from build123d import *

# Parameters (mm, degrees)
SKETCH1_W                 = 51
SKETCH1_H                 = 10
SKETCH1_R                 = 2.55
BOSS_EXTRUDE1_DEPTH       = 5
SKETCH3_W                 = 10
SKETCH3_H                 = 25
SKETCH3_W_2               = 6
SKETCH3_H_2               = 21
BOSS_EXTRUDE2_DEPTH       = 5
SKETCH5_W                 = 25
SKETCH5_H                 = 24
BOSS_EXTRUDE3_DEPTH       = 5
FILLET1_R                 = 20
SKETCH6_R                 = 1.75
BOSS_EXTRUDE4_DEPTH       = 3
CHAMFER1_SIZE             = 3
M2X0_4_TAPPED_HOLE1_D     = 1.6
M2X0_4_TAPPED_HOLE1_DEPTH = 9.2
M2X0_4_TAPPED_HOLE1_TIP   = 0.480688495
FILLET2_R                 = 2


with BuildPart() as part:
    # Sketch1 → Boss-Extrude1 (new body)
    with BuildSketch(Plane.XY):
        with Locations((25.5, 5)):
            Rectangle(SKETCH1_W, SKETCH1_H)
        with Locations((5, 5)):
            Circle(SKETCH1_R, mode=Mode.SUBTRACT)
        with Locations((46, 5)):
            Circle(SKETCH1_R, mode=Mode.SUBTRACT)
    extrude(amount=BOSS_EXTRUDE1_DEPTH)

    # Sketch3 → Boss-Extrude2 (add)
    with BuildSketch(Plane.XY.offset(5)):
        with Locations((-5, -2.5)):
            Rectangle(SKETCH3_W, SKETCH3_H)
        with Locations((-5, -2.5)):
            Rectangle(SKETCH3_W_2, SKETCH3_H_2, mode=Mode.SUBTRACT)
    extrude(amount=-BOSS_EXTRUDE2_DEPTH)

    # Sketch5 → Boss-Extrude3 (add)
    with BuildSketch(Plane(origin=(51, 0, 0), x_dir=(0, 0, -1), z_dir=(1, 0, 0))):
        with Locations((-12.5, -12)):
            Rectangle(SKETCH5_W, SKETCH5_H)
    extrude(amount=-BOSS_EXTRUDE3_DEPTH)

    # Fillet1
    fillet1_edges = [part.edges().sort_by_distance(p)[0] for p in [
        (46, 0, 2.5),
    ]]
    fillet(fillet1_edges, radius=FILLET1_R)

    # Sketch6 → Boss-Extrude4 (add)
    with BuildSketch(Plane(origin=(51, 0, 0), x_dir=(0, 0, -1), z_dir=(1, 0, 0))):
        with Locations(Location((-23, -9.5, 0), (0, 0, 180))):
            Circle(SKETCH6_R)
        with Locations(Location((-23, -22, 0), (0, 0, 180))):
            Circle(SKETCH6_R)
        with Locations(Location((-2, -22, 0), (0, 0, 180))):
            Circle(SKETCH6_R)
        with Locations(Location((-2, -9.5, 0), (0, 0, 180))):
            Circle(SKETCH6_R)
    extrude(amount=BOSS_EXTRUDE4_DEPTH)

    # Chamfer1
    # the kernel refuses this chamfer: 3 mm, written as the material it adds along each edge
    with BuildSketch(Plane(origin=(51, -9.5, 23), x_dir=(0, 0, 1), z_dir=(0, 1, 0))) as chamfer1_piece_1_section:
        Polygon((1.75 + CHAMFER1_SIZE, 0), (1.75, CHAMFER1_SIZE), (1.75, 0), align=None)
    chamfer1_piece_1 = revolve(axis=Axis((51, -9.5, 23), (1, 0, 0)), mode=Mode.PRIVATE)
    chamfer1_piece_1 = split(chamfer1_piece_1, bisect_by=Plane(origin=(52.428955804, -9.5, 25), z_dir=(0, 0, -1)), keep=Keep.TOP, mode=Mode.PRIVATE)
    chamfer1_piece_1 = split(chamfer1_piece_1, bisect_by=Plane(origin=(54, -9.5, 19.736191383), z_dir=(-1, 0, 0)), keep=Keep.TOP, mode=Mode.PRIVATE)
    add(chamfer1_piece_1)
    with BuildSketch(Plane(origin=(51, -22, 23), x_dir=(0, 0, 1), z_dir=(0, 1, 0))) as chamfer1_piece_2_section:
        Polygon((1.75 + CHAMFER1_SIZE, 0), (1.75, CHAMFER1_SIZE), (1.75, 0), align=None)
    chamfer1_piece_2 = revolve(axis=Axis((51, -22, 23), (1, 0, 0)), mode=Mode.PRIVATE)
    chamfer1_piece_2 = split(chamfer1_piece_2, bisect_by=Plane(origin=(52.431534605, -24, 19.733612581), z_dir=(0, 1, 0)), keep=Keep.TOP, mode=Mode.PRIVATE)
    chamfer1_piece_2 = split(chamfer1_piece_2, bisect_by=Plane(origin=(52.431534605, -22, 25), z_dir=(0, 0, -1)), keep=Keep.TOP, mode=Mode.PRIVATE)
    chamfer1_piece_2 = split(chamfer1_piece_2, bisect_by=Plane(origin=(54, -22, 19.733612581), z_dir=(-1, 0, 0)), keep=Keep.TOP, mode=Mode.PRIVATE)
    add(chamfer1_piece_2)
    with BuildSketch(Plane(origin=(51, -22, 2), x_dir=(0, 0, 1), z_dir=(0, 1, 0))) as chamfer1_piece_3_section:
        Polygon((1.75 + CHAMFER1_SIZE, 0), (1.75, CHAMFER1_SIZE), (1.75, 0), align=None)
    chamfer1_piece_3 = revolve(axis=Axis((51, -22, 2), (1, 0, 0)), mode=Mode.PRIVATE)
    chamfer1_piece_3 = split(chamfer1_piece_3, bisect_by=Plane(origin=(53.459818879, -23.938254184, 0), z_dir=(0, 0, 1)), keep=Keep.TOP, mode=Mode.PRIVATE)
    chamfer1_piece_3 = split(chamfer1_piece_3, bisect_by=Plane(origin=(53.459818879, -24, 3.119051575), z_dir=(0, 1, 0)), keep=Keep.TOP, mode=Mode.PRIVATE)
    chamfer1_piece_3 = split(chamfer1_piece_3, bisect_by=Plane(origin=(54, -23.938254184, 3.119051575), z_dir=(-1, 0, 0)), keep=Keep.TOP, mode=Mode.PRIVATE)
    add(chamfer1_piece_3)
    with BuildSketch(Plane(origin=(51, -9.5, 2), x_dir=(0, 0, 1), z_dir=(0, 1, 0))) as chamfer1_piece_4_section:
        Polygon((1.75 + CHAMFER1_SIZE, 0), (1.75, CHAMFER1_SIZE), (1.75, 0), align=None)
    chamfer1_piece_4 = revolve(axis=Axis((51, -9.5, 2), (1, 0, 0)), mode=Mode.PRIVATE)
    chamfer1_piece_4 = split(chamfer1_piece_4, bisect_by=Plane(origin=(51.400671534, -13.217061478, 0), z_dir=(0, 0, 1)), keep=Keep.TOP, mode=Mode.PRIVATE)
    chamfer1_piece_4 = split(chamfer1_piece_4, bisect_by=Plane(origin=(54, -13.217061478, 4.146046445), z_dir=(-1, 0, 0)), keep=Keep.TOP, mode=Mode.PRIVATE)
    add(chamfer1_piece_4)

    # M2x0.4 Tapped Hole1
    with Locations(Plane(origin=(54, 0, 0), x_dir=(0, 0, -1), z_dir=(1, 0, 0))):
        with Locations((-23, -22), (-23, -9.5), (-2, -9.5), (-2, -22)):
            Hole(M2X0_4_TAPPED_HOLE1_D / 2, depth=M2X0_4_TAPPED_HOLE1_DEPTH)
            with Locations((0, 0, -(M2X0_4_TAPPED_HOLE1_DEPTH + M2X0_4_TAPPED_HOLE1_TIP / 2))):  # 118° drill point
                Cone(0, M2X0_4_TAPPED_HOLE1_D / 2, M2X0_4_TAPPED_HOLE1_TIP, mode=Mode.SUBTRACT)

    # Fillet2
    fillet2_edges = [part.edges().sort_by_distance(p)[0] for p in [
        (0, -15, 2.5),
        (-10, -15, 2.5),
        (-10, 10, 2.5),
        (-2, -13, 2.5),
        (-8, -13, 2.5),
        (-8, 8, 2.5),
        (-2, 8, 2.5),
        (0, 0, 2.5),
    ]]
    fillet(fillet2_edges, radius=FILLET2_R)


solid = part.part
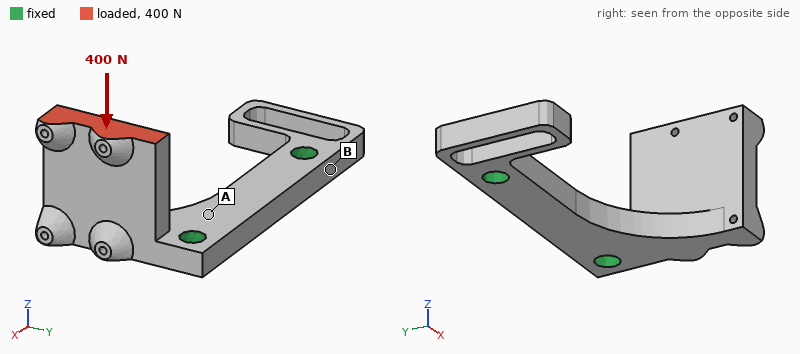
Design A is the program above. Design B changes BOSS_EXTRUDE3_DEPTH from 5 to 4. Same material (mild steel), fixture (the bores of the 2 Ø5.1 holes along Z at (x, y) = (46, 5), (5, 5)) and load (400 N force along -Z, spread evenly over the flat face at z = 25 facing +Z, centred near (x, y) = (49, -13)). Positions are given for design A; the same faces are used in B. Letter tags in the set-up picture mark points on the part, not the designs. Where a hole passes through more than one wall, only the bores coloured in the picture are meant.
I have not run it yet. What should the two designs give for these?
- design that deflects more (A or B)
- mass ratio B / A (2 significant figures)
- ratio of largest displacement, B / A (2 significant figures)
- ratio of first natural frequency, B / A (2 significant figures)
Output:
B
0.91
1.1
1.0
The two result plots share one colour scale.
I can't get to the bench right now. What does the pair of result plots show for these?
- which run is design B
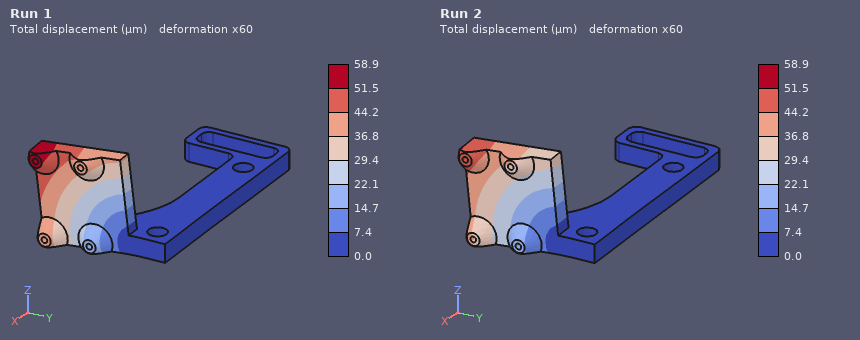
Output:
Run 1
